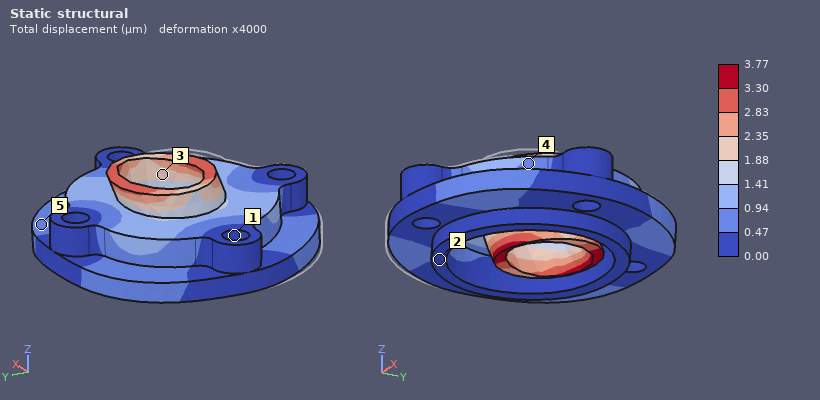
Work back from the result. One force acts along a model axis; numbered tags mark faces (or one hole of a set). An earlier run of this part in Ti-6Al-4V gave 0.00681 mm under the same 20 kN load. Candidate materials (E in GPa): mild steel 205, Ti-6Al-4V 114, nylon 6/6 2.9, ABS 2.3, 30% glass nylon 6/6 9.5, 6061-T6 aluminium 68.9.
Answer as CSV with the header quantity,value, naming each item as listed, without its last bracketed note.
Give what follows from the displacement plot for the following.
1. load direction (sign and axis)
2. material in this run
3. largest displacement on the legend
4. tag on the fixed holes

quantity,value
load direction,+Y
material in this run,mild steel
largest displacement on the legend,3.77 µm
tag on the fixed holes,1
